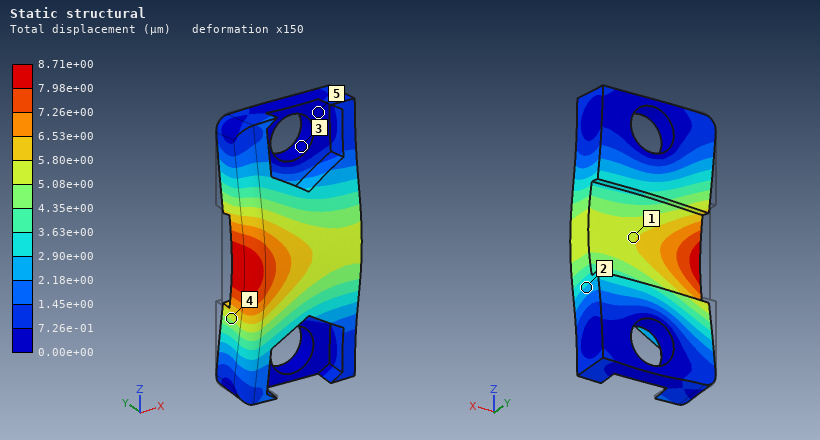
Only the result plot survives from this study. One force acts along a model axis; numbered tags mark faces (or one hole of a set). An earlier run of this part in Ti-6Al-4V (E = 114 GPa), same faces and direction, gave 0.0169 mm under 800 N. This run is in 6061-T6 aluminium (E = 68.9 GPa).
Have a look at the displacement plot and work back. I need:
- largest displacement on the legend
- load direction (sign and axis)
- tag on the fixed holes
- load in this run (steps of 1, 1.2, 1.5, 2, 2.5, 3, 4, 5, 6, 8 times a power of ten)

8.71e+00 µm
-Y
3
250 N
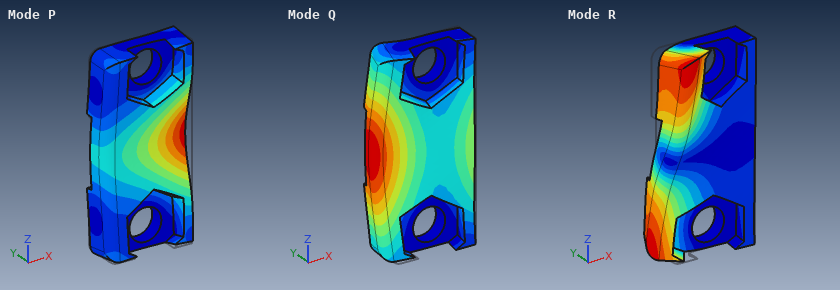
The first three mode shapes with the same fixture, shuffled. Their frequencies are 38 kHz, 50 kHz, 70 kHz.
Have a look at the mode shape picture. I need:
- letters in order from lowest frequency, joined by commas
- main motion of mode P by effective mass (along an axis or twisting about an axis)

Q, P, R
along Y
